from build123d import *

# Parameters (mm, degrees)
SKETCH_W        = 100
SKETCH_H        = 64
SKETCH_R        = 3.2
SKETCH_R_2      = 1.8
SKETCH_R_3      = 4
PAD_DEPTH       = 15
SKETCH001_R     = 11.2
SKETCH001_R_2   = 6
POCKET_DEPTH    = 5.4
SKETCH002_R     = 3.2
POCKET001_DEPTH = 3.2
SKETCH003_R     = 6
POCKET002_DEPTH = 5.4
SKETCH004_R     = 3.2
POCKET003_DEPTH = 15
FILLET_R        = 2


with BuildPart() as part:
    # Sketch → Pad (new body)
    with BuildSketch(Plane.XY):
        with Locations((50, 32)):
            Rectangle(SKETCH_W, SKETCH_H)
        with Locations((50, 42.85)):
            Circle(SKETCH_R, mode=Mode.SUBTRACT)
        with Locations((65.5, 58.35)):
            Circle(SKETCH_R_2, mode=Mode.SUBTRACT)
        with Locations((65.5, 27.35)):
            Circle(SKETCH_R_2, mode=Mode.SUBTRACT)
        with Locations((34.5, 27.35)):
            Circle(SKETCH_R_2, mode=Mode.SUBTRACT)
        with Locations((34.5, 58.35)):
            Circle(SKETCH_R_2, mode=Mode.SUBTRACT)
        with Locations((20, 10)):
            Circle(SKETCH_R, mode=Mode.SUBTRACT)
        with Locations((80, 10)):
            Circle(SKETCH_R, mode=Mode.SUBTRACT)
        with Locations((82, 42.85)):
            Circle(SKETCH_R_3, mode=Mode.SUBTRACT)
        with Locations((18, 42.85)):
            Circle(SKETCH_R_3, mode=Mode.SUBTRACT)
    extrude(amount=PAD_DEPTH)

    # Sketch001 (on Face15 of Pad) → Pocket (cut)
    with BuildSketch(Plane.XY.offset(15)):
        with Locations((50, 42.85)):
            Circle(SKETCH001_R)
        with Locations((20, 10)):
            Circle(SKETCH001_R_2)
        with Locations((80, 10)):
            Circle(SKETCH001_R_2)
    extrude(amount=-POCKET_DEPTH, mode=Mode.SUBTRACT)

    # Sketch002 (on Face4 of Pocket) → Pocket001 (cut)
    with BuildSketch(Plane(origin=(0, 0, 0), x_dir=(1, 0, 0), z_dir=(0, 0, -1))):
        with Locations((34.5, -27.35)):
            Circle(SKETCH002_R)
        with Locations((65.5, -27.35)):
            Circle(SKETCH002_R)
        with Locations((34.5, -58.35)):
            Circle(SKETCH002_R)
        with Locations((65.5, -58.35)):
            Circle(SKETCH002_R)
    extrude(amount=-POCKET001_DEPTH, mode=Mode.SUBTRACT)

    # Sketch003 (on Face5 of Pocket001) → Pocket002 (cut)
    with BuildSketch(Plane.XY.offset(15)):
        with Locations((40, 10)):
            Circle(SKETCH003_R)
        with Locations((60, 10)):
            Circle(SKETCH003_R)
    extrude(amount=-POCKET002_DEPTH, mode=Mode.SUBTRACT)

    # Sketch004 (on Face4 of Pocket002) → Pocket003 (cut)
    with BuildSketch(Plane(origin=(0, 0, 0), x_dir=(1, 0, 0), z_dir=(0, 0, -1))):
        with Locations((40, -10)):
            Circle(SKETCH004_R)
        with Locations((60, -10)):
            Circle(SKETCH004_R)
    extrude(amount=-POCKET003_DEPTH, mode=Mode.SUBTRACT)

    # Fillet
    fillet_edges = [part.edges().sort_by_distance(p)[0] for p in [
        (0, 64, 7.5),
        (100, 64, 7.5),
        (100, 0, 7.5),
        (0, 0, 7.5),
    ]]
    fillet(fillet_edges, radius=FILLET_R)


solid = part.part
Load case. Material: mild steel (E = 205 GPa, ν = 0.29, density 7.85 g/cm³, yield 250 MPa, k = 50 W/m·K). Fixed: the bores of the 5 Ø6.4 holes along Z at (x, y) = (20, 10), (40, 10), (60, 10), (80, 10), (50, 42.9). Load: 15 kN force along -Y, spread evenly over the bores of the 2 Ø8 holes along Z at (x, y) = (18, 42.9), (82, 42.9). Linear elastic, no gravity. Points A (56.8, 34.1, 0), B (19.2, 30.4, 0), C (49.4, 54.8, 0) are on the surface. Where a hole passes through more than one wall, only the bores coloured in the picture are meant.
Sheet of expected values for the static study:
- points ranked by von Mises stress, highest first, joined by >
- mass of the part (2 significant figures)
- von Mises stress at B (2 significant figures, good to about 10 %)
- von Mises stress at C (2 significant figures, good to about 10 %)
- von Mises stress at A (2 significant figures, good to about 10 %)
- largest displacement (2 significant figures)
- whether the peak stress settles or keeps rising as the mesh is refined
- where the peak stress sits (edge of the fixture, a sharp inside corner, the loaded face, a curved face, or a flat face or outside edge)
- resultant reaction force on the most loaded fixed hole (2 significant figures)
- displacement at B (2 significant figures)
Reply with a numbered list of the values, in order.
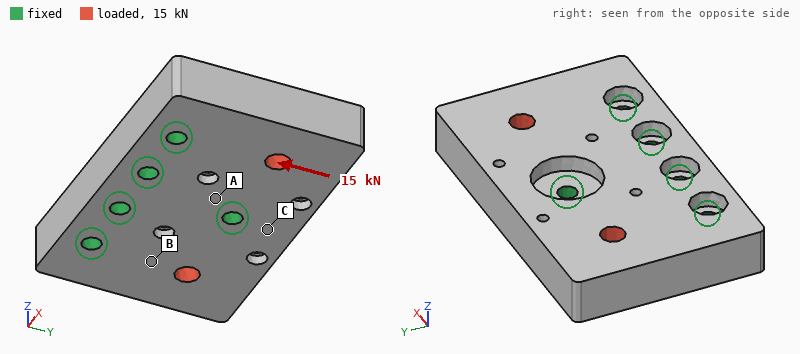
1. B > C > A
2. 690 g
3. 20 MPa
4. 13 MPa
5. 5.0 MPa
6. 4.1 µm
7. keeps rising
8. edge of the fixture
9. 4.5 kN
10. 1.9 µm
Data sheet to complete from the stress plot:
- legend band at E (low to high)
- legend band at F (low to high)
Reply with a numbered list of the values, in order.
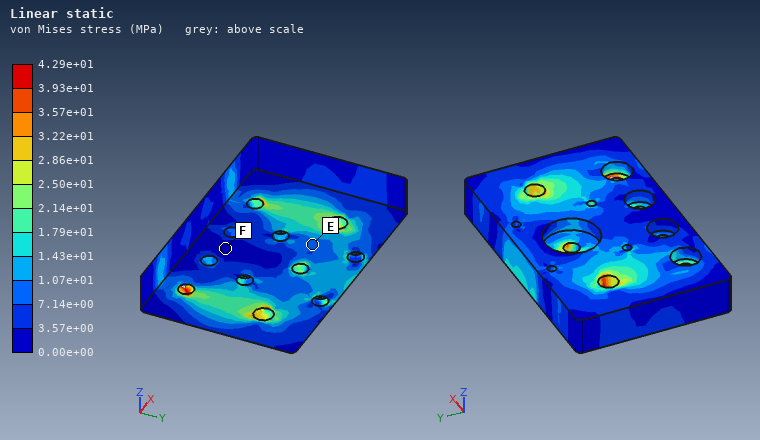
1. 7.14e+00 to 1.07e+01 MPa
2. 0.00e+00 to 3.57e+00 MPa
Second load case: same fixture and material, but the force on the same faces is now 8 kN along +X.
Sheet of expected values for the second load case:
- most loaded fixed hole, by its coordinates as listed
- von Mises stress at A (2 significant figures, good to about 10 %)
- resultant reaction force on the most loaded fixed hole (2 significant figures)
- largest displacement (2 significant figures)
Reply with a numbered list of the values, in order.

1. (50, 42.9)
2. 4.2 MPa
3. 5.4 kN
4. 3.2 µm
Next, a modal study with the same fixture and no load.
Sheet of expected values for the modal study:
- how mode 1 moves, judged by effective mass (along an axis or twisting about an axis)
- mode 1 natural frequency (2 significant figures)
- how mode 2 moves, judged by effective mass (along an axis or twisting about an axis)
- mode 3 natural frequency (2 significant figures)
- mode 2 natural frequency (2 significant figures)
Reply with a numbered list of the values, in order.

1. twisting about Y
2. 5200 Hz
3. along Z
4. 13 kHz
5. 5800 Hz
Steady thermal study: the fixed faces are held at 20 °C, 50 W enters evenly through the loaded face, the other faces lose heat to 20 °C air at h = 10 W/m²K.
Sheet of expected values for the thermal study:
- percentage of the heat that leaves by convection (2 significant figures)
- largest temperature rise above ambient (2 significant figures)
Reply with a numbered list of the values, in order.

1. 3.8 %
2. 25 K
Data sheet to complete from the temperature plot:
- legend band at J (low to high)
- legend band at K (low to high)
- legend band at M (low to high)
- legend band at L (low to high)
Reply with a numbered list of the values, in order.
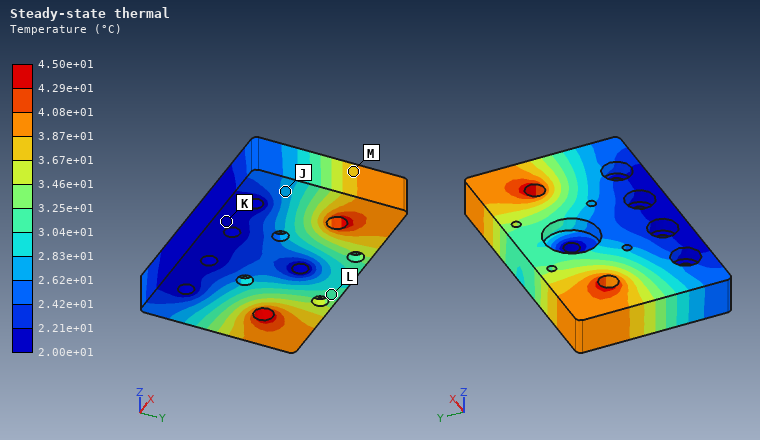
1. 2.62e+01 to 2.83e+01 °C
2. 2.00e+01 to 2.21e+01 °C
3. 3.67e+01 to 3.87e+01 °C
4. 3.04e+01 to 3.25e+01 °C
